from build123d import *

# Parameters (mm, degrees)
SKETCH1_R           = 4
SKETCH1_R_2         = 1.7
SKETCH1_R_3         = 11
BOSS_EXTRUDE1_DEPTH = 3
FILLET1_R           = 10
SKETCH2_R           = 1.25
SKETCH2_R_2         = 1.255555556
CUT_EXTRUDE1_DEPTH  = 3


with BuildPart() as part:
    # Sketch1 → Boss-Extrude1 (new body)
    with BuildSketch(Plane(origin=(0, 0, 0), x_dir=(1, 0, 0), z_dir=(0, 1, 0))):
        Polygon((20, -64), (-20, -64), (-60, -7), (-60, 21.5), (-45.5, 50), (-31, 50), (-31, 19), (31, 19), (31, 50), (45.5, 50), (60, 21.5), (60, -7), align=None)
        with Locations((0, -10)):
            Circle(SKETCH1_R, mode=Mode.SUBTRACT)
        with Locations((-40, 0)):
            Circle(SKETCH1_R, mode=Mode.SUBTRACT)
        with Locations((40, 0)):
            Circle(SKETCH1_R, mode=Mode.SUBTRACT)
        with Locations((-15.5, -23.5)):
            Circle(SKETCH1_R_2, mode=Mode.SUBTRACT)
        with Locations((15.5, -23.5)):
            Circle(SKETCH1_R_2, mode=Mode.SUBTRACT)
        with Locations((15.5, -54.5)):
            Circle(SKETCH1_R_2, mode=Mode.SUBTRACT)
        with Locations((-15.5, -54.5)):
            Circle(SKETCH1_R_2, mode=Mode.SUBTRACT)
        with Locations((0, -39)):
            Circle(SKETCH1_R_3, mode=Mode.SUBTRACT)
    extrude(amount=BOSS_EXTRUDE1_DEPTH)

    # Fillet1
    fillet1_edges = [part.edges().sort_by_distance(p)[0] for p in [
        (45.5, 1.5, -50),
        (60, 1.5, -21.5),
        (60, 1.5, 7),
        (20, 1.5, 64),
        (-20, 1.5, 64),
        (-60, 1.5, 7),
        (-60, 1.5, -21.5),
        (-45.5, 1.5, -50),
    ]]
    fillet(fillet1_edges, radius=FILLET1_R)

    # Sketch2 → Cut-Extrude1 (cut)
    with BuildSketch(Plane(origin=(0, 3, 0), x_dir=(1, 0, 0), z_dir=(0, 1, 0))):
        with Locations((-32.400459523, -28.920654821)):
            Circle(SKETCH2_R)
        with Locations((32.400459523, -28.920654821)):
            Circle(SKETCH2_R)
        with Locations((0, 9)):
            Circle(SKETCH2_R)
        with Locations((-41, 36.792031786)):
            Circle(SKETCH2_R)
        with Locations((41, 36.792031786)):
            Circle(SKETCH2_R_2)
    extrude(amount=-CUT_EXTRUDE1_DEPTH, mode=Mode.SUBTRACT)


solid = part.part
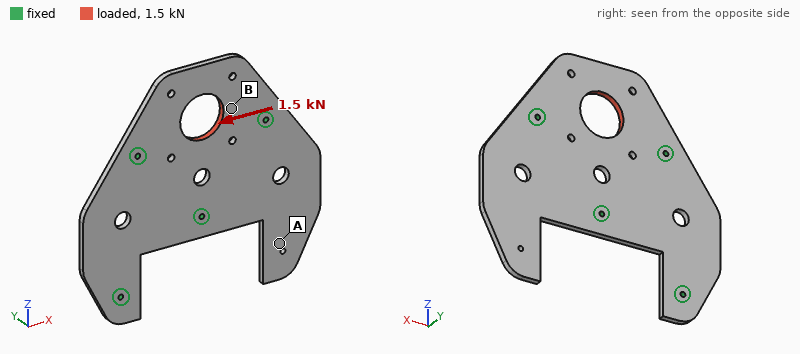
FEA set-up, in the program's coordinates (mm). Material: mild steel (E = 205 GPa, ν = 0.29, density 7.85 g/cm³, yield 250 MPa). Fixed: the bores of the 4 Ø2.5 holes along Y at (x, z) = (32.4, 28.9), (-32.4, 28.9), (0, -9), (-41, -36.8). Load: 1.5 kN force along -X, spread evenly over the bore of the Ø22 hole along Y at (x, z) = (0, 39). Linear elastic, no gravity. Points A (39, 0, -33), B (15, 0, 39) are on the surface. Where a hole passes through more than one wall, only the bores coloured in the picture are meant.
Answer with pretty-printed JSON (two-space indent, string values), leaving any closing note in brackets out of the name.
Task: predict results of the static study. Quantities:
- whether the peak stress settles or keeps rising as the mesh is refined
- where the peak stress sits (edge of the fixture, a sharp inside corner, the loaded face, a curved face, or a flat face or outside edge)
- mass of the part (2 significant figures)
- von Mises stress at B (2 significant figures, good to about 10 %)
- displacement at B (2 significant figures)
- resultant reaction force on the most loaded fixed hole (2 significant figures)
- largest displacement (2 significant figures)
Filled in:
{
  "whether the peak stress settles or keeps rising as the mesh is refined": "keeps rising",
  "where the peak stress sits": "edge of the fixture",
  "mass of the part": "200 g",
  "von Mises stress at B": "12 MPa",
  "displacement at B": "1.9 µm",
  "resultant reaction force on the most loaded fixed hole": "750 N",
  "largest displacement": "3.3 µm"
}
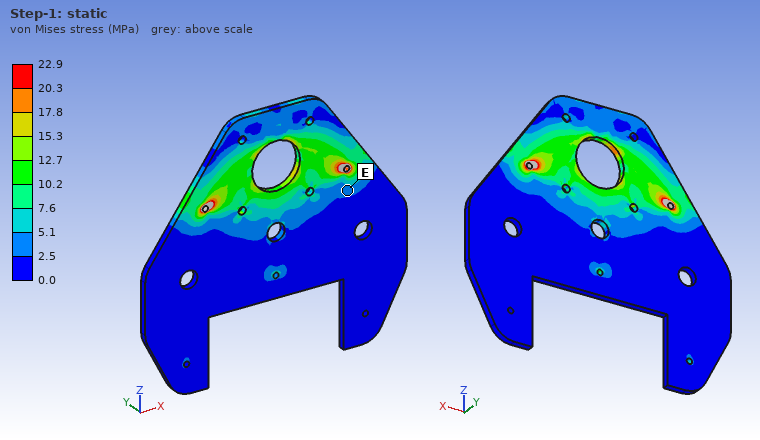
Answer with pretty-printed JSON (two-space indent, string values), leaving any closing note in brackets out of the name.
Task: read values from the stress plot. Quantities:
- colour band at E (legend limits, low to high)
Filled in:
{
  "colour band at E": "2.5 to 5.1 MPa"
}
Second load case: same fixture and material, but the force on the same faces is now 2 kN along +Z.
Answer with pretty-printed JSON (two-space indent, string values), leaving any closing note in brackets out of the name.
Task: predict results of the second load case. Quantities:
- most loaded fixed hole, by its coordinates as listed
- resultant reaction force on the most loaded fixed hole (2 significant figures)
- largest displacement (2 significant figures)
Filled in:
{
  "most loaded fixed hole, by its coordinates as listed": "(32.4, 28.9)",
  "resultant reaction force on the most loaded fixed hole": "740 N",
  "largest displacement": "3.7 µm"
}
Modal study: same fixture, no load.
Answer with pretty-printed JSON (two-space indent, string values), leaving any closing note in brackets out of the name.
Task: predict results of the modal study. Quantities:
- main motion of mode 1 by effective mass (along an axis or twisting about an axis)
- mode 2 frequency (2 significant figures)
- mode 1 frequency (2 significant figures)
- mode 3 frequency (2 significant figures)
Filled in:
{
  "main motion of mode 1 by effective mass": "along Y",
  "mode 2 frequency": "1600 Hz",
  "mode 1 frequency": "720 Hz",
  "mode 3 frequency": "2100 Hz"
}
